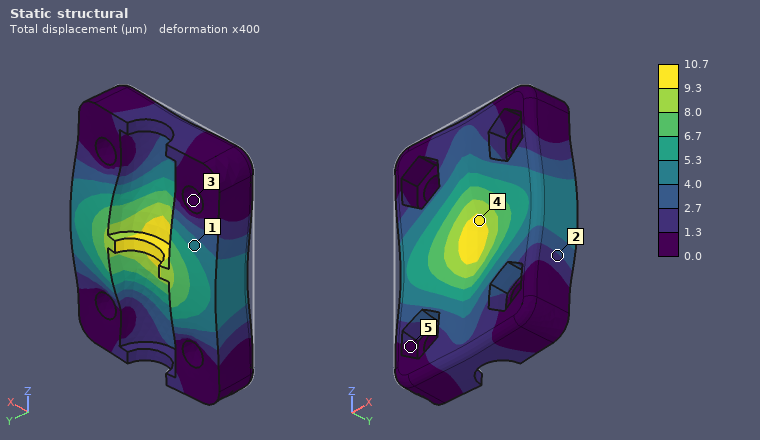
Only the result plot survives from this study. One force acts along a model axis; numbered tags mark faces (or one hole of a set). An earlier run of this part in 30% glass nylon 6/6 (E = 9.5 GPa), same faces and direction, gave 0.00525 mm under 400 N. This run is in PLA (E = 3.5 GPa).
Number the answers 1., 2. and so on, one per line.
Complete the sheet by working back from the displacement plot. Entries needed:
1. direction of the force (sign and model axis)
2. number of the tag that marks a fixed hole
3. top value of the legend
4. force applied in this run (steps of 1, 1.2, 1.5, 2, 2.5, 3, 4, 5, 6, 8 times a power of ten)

1. +Y
2. 3
3. 10.7 µm
4. 300 N
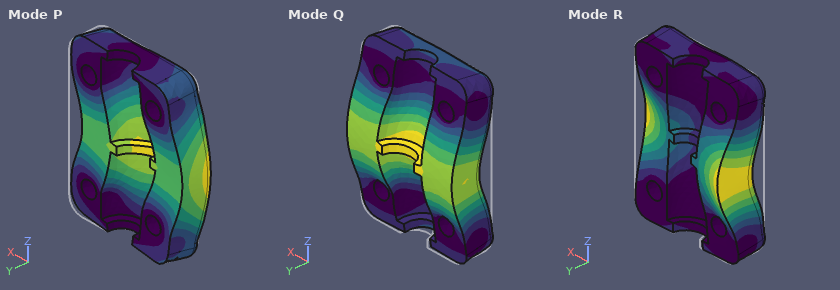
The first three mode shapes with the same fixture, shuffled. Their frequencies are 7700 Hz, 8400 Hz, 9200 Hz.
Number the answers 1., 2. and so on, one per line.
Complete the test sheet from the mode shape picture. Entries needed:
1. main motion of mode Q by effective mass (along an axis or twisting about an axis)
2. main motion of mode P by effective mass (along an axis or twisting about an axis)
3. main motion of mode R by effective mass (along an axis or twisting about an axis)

1. along Y
2. along X
3. twisting about Z
